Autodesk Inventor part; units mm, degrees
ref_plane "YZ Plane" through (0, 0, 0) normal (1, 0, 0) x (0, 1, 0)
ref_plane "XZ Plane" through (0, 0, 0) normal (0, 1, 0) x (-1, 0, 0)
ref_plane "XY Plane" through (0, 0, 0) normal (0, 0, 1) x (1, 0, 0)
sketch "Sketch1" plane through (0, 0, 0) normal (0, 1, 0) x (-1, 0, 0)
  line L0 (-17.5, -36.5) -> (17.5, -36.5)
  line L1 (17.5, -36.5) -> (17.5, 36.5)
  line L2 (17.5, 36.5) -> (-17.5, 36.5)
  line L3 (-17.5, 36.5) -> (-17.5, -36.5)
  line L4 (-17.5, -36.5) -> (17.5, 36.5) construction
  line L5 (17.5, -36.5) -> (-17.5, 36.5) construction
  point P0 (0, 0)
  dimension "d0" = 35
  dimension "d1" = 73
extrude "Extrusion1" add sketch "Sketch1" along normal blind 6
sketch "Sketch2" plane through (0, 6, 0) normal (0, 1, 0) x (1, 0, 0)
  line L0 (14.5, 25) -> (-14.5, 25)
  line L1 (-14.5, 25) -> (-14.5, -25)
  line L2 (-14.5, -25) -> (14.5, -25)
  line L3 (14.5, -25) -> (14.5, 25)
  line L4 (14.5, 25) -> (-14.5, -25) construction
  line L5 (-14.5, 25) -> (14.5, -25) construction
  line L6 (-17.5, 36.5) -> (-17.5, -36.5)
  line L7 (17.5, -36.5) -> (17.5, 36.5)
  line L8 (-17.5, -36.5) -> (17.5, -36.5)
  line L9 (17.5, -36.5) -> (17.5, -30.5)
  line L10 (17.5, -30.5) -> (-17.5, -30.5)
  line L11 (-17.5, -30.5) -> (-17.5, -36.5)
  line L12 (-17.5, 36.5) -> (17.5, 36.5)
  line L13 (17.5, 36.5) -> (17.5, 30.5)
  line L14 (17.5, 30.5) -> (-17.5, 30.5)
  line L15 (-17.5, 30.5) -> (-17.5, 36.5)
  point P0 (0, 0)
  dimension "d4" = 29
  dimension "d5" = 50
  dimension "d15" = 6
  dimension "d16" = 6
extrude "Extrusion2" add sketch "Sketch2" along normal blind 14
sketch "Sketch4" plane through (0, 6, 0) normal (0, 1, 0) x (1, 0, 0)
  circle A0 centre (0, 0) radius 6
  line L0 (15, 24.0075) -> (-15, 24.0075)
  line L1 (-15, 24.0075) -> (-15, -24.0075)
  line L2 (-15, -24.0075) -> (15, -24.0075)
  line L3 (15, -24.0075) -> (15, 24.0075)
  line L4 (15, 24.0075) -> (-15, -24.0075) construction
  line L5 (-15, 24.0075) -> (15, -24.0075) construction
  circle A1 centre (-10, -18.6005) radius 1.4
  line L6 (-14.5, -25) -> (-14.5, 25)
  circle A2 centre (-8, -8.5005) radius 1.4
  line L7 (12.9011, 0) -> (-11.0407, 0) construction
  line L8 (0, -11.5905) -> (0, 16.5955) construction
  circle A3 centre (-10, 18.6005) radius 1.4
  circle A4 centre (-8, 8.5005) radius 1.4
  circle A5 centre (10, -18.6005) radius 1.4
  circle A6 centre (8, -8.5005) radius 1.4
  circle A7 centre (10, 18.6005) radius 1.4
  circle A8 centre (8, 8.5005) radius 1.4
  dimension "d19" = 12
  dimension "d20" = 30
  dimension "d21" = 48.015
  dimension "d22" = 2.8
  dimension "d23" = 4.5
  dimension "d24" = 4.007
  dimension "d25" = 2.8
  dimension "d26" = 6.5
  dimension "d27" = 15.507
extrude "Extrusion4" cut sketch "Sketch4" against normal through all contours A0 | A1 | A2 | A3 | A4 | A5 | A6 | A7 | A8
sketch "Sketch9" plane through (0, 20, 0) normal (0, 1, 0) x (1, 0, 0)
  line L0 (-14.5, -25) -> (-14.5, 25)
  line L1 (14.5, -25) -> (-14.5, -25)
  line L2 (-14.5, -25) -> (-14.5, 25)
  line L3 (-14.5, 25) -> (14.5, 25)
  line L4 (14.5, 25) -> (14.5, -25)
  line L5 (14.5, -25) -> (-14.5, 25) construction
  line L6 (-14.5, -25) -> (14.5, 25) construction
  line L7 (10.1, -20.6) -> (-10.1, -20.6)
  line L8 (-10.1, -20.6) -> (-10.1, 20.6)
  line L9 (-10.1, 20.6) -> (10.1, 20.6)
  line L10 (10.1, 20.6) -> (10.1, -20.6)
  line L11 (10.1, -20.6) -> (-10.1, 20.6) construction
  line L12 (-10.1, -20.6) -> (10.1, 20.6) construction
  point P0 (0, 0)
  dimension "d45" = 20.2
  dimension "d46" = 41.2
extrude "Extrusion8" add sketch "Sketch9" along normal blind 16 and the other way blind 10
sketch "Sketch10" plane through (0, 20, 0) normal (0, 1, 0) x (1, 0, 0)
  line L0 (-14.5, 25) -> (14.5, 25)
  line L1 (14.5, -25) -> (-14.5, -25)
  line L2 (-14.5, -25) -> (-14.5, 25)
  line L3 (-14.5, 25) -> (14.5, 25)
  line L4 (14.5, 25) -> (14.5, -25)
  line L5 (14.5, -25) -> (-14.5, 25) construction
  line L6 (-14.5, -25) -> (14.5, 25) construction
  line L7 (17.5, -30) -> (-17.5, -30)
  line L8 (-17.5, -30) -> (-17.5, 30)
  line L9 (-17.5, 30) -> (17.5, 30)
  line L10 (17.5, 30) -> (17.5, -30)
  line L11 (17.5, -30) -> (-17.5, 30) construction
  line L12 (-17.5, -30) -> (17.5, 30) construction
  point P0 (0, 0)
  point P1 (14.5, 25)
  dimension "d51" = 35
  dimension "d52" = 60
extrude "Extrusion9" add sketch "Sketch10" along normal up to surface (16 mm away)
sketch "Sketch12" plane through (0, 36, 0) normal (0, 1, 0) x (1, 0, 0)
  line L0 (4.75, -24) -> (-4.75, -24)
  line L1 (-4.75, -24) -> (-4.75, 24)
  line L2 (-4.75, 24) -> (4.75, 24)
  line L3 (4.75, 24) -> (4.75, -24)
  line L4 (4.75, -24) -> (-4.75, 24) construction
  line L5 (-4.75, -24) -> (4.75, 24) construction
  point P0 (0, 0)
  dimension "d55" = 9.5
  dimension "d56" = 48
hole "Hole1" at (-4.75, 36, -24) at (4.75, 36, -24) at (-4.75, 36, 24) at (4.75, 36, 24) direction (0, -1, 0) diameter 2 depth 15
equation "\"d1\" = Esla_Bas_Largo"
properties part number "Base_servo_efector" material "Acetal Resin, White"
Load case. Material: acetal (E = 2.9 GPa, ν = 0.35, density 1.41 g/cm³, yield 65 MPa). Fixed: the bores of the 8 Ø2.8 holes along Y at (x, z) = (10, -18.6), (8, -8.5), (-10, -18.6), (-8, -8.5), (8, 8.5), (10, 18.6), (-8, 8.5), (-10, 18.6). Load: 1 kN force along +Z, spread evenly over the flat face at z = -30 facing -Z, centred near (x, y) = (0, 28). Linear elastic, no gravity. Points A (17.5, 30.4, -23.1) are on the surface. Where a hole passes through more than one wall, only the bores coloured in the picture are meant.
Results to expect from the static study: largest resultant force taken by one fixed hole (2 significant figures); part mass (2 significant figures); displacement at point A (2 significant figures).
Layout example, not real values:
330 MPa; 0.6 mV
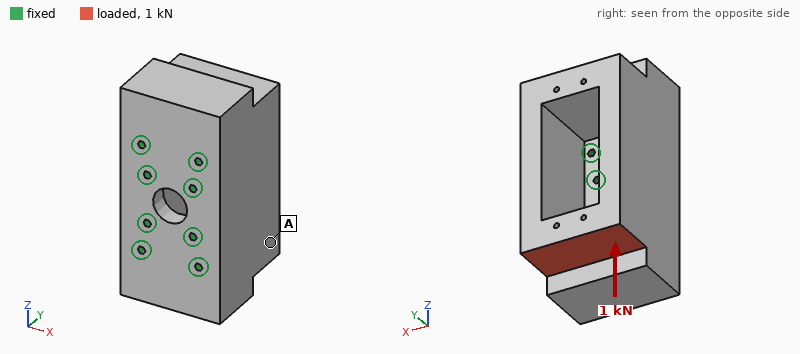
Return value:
330 N; 79 g; 0.12 mm
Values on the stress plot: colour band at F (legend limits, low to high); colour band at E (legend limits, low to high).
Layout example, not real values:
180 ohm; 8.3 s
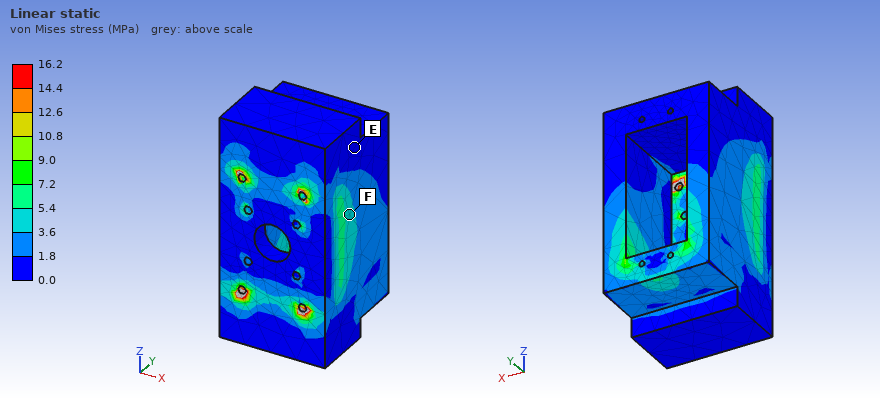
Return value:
3.6 to 5.4 MPa; 0.0 to 1.8 MPa
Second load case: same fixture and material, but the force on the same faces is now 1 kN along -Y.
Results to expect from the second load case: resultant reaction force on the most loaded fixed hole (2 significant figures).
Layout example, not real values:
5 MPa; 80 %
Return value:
560 N
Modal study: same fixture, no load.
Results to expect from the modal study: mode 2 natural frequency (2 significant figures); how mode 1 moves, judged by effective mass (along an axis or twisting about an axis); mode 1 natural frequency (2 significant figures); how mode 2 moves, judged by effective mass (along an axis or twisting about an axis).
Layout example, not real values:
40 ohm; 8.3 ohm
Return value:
2100 Hz; along X; 1900 Hz; along Z
